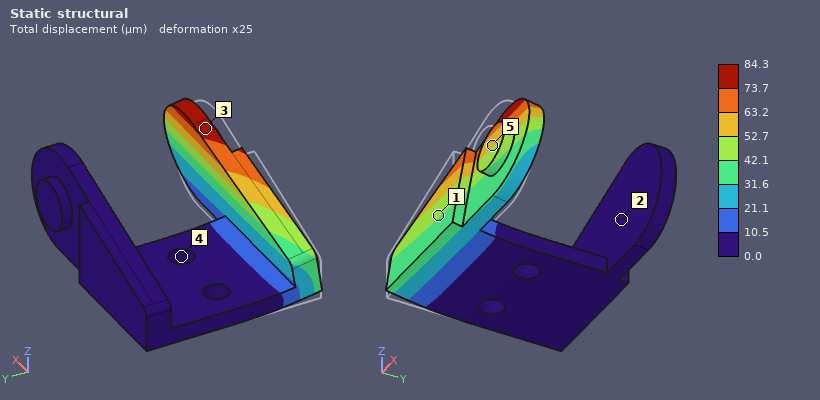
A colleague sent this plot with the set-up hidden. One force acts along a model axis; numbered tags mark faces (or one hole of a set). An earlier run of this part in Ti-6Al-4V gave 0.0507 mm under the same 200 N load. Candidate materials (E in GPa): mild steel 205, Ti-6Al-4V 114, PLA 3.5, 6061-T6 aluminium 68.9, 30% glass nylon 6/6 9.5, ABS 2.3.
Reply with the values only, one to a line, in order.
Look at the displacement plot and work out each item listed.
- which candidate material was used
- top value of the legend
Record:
6061-T6 aluminium
84.3 µm
